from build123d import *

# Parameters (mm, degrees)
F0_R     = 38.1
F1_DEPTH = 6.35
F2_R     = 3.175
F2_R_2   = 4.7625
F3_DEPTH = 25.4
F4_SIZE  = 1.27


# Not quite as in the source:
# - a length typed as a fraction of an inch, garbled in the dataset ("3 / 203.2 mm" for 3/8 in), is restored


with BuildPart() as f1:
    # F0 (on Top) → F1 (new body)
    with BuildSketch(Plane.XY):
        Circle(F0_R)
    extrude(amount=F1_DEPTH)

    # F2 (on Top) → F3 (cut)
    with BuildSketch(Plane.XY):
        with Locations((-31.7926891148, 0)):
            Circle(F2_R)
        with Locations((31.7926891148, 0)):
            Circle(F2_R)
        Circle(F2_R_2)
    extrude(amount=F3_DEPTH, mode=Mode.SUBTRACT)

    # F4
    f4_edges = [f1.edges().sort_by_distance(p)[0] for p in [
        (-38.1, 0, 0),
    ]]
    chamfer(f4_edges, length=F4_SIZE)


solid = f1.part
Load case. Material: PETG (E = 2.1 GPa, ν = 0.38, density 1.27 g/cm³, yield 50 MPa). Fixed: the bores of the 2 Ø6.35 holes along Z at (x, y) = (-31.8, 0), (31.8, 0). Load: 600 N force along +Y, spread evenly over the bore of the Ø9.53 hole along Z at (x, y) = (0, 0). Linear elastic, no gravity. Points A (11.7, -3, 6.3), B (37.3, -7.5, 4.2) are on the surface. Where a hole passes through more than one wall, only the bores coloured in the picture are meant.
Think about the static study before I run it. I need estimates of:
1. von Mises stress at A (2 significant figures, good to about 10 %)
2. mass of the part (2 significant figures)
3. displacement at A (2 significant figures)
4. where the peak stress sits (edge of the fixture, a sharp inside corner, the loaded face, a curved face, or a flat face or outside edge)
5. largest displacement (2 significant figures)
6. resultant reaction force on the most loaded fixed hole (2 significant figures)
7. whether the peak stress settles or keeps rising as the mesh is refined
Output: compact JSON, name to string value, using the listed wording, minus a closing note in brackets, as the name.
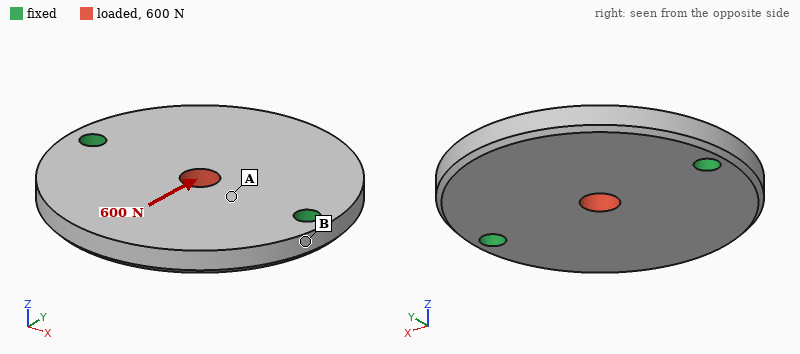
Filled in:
{"von Mises stress at A": "1.4 MPa", "mass of the part": "35 g", "displacement at A": "35 µm", "where the peak stress sits": "edge of the fixture", "largest displacement": "53 µm", "resultant reaction force on the most loaded fixed hole": "300 N", "whether the peak stress settles or keeps rising as the mesh is refined": "keeps rising"}
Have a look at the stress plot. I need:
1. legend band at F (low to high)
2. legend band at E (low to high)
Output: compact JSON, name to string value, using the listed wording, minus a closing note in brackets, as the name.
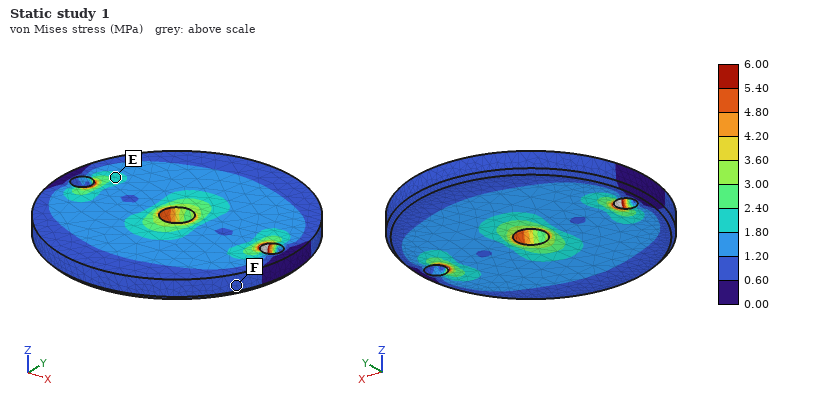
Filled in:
{"legend band at F": "0.60 to 1.20 MPa", "legend band at E": "1.80 to 2.40 MPa"}
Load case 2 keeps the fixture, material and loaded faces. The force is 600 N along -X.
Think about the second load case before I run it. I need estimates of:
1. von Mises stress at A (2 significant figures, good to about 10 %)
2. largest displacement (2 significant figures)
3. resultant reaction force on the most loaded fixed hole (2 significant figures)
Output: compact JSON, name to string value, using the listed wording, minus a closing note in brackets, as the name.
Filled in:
{"von Mises stress at A": "2.6 MPa", "largest displacement": "36 µm", "resultant reaction force on the most loaded fixed hole": "300 N"}
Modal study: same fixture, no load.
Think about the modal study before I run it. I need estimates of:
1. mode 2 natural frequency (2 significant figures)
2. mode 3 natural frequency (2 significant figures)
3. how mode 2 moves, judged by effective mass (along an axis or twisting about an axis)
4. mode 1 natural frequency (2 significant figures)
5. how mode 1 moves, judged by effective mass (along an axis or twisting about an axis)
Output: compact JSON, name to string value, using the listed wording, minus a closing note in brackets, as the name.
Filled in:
{"mode 2 natural frequency": "1000 Hz", "mode 3 natural frequency": "2200 Hz", "how mode 2 moves, judged by effective mass": "along Z", "mode 1 natural frequency": "770 Hz", "how mode 1 moves, judged by effective mass": "twisting about X"}
